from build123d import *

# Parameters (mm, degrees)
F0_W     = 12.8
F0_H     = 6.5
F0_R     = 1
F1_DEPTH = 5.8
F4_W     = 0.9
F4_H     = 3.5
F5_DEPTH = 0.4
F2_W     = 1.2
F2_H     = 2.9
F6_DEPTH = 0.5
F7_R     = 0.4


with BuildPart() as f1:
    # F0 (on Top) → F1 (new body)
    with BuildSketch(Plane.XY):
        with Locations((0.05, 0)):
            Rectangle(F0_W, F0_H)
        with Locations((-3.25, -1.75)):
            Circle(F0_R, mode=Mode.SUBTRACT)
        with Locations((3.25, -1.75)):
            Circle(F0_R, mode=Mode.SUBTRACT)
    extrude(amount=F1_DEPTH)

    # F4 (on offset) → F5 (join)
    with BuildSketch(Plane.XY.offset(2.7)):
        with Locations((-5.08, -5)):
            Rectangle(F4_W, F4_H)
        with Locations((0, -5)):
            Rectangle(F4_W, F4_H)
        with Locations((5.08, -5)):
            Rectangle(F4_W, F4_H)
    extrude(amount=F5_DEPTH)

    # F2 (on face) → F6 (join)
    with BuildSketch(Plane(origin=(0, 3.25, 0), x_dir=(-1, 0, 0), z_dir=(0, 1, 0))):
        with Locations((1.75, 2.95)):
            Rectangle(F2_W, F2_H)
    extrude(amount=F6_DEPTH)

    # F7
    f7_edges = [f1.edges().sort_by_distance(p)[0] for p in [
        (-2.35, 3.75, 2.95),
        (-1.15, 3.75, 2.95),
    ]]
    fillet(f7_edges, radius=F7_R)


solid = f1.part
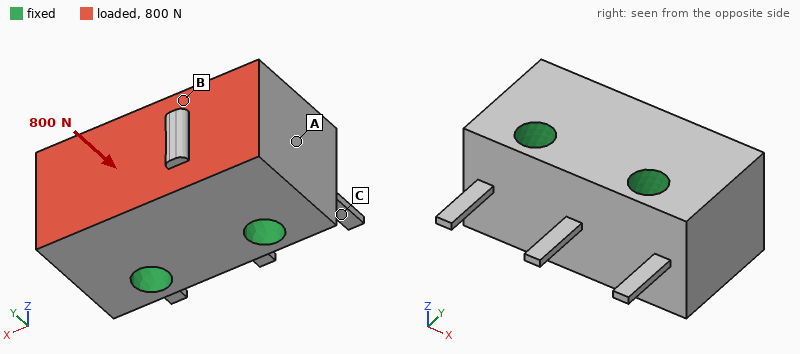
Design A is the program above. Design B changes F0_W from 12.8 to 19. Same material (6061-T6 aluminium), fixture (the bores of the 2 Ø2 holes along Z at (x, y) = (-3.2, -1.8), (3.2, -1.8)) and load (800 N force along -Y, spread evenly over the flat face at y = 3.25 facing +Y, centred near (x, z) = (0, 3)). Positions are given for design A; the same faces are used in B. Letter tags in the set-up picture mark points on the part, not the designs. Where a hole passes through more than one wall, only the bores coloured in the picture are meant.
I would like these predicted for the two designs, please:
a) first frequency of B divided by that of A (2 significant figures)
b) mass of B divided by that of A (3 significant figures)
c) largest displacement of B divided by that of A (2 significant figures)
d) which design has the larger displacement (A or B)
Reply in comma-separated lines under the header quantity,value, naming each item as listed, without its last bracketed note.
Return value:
quantity,value
first frequency of B divided by that of A,1.0
mass of B divided by that of A,1.52
largest displacement of B divided by that of A,2.5
which design has the larger displacement,B
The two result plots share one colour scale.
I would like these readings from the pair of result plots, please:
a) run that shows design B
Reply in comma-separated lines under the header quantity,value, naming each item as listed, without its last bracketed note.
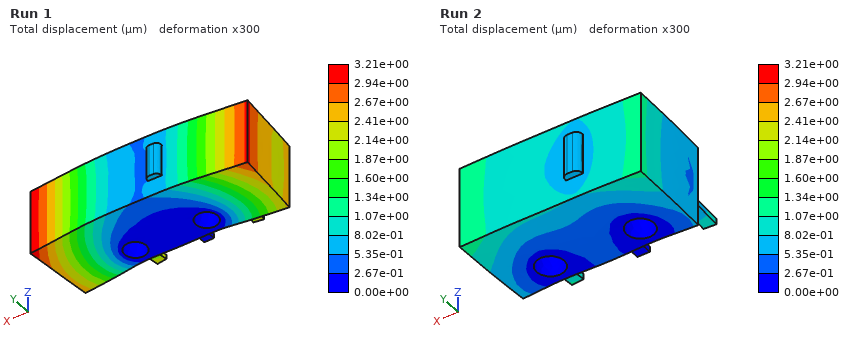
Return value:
quantity,value
run that shows design B,Run 1
